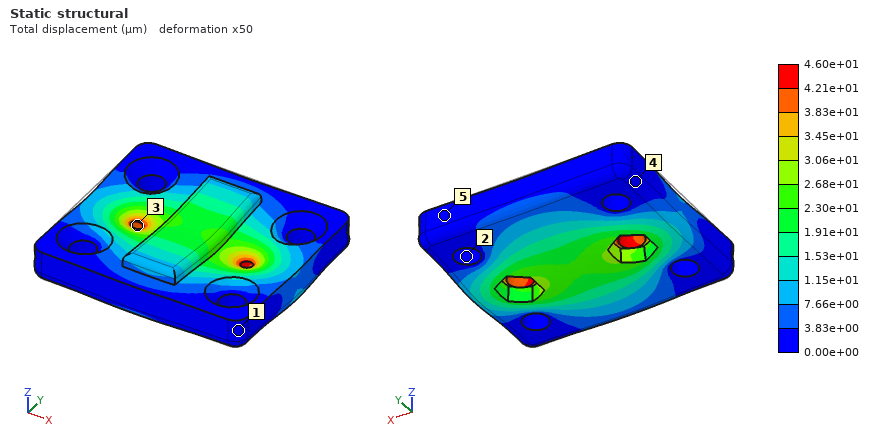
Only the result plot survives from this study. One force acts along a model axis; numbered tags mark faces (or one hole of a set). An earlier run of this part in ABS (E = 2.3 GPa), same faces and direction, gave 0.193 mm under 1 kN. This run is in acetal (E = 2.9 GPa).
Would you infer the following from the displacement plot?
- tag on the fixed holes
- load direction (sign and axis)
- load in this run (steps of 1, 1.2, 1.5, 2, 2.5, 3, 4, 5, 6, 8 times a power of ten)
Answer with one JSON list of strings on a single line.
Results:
["2", "-Z", "300 N"]
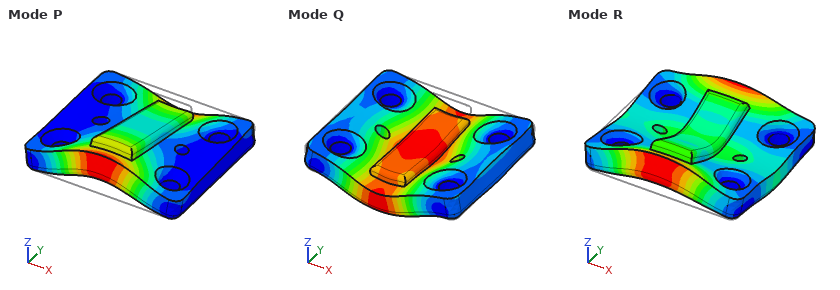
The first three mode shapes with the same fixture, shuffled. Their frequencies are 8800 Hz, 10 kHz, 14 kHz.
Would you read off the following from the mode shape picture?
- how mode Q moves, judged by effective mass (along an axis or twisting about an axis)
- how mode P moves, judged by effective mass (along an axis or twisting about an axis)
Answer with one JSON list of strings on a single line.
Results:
["along Z", "twisting about X"]
